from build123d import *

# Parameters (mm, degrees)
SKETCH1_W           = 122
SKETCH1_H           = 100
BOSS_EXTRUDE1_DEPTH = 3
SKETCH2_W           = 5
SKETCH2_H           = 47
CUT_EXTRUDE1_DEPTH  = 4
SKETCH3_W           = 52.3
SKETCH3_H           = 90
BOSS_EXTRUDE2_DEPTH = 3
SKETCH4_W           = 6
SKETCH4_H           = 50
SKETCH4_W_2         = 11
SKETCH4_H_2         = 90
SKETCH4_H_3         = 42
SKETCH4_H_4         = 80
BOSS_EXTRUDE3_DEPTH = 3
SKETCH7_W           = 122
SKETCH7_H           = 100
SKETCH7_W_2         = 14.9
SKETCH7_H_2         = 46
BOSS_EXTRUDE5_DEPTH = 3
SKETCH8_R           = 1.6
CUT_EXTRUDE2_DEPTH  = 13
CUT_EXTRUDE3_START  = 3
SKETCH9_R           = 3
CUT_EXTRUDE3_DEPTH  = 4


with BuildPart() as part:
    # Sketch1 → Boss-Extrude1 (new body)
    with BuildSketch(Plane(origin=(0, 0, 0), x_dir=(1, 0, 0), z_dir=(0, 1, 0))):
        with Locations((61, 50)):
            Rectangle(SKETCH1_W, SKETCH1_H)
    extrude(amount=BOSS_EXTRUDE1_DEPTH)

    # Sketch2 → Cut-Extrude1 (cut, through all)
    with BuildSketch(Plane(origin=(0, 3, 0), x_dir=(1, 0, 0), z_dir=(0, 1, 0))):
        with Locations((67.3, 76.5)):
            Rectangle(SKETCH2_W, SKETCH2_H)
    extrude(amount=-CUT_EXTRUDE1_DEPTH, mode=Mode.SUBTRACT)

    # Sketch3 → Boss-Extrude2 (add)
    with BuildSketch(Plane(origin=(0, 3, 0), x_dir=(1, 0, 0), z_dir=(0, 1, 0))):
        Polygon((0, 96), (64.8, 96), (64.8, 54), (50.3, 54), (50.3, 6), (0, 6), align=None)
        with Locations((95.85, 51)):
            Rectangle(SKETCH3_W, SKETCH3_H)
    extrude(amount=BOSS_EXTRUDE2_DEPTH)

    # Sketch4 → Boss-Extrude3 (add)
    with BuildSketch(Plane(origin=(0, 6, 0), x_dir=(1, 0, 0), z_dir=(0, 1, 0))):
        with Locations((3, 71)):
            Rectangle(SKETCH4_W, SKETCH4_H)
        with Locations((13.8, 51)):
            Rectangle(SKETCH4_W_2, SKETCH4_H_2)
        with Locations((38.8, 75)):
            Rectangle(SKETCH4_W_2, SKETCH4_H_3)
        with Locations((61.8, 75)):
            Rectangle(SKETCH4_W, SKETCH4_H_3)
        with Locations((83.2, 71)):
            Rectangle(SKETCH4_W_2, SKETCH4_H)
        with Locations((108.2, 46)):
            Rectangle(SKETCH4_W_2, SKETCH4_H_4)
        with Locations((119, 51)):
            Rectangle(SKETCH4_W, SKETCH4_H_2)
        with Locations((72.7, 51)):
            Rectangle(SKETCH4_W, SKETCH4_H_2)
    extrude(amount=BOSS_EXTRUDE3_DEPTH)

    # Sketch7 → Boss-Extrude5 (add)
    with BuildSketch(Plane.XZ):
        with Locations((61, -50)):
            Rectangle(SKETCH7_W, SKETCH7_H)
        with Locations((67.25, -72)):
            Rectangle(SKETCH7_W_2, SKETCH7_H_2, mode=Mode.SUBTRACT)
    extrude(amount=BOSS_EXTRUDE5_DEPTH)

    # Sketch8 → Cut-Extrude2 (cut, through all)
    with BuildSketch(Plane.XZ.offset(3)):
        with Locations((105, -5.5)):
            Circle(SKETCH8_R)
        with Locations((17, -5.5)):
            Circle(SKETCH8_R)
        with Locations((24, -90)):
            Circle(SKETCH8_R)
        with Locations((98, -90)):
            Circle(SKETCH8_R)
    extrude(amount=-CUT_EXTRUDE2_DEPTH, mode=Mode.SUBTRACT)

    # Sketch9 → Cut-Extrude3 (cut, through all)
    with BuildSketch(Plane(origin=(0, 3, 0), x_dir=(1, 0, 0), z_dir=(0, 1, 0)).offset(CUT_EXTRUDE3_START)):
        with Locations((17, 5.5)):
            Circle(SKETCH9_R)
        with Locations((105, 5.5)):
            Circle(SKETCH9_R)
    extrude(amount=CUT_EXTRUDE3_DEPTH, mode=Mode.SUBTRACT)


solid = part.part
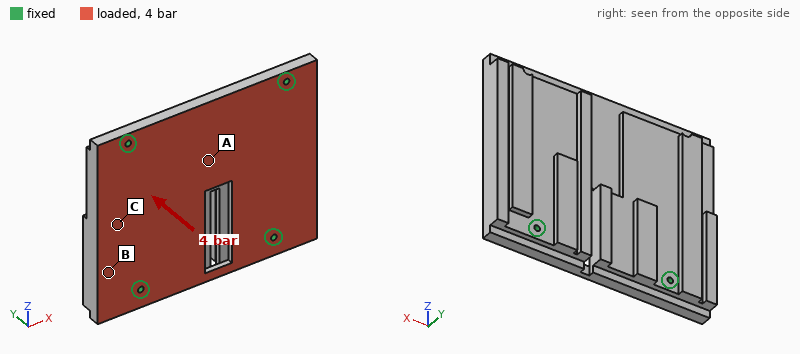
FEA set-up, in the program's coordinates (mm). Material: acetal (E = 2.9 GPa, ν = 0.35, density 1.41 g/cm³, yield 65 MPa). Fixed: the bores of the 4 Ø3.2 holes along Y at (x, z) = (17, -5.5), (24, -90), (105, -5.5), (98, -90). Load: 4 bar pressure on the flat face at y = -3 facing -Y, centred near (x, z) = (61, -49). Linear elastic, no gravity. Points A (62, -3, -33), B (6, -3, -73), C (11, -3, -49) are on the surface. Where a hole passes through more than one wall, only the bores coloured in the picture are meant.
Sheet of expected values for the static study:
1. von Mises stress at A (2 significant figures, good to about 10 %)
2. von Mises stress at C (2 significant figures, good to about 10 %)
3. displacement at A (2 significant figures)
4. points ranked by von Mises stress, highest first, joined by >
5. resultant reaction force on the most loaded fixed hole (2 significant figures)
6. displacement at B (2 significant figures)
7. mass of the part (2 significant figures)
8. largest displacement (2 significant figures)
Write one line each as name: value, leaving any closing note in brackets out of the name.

von Mises stress at A: 18 MPa
von Mises stress at C: 11 MPa
displacement at A: 1.2 mm
points ranked by von Mises stress, highest first, joined by >: A > C > B
resultant reaction force on the most loaded fixed hole: 1.3 kN
displacement at B: 0.22 mm
mass of the part: 160 g
largest displacement: 1.3 mm
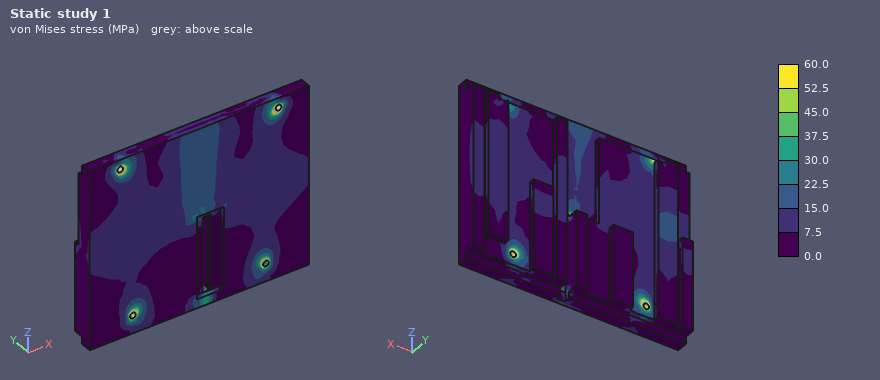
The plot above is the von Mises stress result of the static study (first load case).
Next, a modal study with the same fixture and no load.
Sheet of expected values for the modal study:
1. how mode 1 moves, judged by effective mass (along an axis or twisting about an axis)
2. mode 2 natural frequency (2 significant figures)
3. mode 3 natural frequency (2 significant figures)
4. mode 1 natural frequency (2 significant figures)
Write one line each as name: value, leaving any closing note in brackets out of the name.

how mode 1 moves, judged by effective mass: along Y
mode 2 natural frequency: 1400 Hz
mode 3 natural frequency: 1400 Hz
mode 1 natural frequency: 920 Hz
